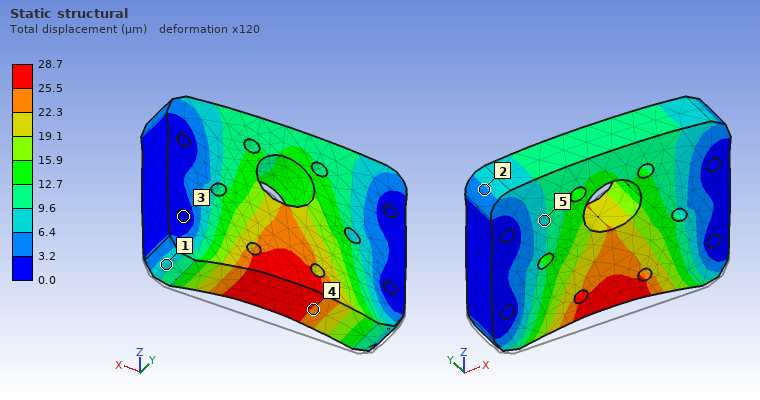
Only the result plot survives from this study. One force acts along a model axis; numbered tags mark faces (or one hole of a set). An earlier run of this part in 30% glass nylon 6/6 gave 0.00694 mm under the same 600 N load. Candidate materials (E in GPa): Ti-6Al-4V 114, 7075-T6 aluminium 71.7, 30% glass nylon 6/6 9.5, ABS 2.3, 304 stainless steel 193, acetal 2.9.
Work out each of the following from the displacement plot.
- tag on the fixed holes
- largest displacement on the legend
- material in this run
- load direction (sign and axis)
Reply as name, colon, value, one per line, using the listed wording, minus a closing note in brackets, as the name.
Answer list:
tag on the fixed holes: 3
largest displacement on the legend: 28.7 µm
material in this run: ABS
load direction: +Z
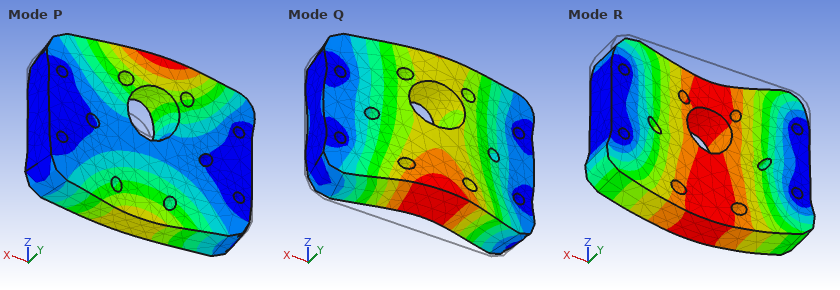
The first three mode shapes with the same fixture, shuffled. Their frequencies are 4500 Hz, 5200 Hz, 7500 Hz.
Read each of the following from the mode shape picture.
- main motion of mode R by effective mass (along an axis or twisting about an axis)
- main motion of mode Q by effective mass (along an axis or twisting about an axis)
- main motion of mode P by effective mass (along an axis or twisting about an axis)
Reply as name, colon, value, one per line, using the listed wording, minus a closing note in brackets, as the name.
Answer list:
main motion of mode R by effective mass: along Z
main motion of mode Q by effective mass: along Y
main motion of mode P by effective mass: twisting about X
